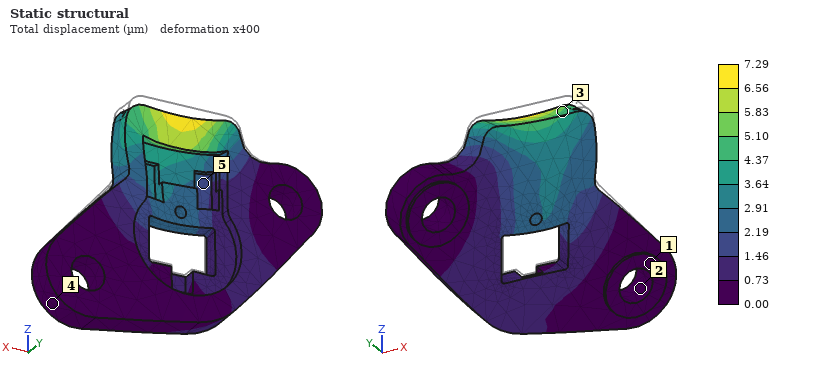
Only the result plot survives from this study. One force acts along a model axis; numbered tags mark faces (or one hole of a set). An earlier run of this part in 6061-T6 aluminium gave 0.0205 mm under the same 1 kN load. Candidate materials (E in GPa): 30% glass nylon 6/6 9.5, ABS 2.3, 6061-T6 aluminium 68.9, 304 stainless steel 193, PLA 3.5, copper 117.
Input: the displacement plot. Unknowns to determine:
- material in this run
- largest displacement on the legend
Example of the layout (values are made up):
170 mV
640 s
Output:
304 stainless steel
7.29 µm
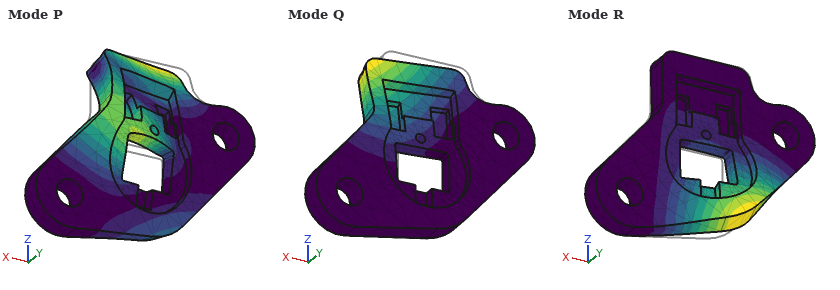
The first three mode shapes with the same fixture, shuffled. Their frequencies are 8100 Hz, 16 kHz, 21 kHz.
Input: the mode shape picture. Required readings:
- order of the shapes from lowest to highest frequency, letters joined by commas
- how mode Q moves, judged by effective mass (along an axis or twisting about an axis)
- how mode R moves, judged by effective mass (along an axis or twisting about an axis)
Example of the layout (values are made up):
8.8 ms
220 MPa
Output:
Q, R, P
along Y
along Y
